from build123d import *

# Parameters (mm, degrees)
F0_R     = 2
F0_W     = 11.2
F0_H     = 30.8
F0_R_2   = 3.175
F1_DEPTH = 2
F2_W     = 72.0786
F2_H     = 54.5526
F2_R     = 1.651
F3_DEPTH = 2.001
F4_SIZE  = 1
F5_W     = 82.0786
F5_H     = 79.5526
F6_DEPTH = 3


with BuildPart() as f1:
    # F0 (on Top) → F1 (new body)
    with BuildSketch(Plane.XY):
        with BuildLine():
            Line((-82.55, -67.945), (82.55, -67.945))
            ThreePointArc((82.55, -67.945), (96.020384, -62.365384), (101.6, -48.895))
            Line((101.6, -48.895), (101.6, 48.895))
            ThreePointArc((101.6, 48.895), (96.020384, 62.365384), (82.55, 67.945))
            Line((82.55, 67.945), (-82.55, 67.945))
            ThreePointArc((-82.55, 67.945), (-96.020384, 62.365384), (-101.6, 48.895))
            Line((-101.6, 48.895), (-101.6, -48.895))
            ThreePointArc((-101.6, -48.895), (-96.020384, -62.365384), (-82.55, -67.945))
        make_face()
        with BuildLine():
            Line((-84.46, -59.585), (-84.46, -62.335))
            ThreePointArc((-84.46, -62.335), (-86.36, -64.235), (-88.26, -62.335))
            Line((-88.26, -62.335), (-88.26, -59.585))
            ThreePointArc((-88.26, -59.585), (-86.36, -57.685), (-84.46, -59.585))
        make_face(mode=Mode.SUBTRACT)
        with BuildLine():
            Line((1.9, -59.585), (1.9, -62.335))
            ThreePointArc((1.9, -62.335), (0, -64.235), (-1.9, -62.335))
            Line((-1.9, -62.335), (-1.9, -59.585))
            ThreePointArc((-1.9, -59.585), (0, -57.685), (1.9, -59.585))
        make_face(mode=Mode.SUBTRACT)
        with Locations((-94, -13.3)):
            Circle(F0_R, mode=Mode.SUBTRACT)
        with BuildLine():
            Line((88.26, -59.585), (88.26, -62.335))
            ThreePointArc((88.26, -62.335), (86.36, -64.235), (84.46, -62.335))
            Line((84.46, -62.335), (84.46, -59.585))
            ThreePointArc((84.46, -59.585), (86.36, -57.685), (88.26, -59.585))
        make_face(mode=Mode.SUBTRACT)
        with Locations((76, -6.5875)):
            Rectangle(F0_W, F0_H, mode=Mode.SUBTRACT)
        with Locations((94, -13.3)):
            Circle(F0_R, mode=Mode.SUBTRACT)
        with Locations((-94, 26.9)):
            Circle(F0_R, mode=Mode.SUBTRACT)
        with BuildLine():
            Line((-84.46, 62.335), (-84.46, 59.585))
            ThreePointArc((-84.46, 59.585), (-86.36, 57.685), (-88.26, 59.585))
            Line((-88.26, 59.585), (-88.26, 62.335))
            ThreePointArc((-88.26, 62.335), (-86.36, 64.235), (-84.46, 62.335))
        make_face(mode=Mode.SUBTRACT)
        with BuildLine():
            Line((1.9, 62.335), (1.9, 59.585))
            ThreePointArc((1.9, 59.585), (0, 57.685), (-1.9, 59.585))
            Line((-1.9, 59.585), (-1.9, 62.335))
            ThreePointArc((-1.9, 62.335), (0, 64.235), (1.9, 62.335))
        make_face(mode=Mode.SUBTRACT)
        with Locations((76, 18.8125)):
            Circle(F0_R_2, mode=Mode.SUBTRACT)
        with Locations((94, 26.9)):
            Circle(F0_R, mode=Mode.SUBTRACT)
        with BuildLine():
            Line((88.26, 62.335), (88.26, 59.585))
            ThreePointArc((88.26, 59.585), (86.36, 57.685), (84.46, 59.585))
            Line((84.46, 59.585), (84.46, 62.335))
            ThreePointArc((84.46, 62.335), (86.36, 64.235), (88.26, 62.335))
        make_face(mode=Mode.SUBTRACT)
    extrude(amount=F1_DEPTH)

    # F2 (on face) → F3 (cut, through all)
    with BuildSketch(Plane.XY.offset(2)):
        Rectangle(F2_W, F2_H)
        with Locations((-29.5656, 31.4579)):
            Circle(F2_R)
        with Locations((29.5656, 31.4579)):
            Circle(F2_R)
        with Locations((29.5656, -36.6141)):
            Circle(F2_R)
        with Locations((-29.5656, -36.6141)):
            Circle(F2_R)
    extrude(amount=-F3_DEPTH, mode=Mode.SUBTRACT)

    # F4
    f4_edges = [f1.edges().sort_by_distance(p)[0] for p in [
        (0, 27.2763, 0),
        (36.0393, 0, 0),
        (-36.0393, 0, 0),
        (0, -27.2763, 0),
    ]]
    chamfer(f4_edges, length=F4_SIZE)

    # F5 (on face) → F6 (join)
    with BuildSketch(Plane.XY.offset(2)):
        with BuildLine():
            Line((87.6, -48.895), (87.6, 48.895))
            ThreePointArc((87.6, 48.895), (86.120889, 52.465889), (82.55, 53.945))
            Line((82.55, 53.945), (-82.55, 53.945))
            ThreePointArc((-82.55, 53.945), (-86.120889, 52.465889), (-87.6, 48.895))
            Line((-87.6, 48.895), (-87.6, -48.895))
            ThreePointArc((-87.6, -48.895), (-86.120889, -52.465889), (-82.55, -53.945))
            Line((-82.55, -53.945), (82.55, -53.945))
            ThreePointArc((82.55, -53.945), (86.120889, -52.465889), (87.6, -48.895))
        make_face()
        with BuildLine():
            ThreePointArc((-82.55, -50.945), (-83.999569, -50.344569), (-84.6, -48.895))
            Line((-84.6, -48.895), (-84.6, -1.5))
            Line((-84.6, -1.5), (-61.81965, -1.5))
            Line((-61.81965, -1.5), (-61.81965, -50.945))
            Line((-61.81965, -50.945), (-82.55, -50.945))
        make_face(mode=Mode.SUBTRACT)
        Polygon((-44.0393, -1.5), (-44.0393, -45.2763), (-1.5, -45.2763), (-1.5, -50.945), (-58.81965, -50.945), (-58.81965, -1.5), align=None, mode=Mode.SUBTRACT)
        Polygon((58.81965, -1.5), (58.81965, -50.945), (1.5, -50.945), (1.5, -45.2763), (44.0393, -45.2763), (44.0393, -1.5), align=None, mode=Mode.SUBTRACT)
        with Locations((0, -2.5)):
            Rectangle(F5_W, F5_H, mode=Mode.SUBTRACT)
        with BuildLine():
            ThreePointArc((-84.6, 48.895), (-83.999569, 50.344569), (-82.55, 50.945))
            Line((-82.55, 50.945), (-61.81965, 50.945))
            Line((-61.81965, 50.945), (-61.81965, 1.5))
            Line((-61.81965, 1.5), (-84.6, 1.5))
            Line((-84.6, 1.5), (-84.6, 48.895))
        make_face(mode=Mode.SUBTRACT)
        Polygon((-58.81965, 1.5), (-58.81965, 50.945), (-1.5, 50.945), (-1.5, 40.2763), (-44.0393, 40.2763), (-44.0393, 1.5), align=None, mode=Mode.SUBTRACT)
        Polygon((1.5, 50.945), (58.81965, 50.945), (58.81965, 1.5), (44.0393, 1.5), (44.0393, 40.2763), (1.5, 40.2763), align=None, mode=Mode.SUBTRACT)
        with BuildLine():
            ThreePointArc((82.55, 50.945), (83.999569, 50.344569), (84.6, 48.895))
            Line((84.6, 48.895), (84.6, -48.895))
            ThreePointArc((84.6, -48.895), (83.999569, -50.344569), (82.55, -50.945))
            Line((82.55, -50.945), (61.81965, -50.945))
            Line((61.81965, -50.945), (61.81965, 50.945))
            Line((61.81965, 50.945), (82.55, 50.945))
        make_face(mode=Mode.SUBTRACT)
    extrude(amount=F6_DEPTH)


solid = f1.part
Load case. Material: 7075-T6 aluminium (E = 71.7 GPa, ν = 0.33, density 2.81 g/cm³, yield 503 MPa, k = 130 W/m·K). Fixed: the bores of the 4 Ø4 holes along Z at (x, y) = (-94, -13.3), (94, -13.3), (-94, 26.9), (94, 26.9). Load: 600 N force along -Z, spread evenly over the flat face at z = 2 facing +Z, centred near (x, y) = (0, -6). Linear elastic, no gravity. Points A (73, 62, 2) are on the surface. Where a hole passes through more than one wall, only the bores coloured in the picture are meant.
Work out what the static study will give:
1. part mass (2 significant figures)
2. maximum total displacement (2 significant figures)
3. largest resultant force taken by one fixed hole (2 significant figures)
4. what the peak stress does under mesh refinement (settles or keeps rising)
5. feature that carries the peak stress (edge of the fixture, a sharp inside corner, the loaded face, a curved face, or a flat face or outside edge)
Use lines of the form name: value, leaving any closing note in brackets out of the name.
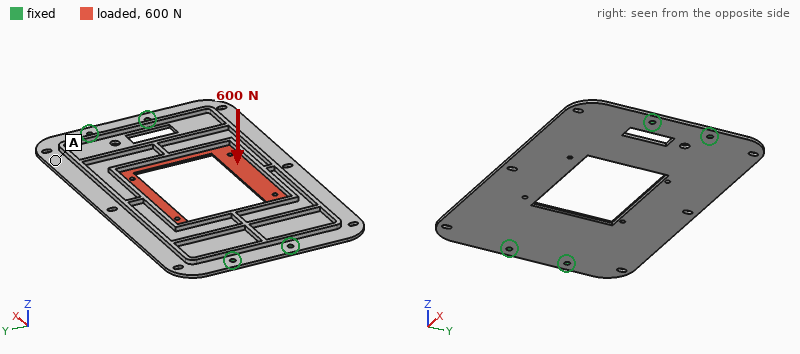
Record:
part mass: 160 g
maximum total displacement: 2.5 mm
largest resultant force taken by one fixed hole: 550 N
what the peak stress does under mesh refinement: keeps rising
feature that carries the peak stress: edge of the fixture
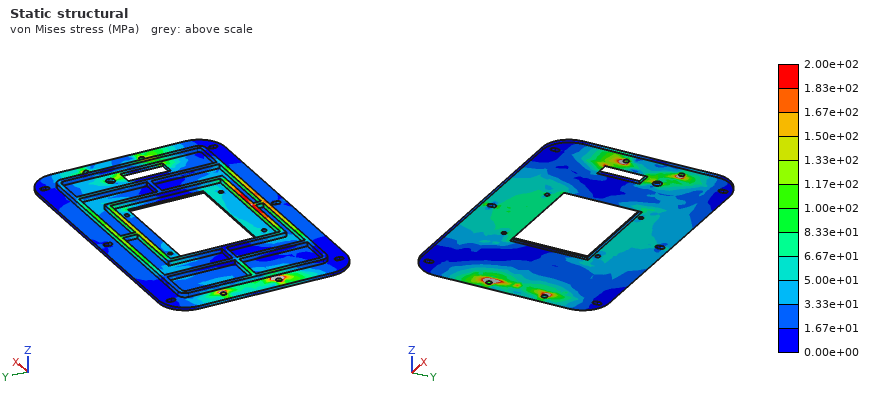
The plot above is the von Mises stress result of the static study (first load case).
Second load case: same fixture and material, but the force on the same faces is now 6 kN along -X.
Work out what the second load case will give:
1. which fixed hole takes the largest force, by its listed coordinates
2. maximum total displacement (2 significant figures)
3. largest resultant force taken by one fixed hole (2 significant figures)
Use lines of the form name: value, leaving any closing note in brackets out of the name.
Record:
which fixed hole takes the largest force, by its listed coordinates: (-94, -13.3)
maximum total displacement: 68 µm
largest resultant force taken by one fixed hole: 2.2 kN
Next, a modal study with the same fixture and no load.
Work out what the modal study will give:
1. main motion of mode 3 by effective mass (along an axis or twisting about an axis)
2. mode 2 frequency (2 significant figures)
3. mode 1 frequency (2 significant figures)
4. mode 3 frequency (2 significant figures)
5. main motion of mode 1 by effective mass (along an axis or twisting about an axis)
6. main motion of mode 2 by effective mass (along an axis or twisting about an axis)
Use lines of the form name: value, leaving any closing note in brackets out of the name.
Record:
main motion of mode 3 by effective mass: twisting about Y
mode 2 frequency: 380 Hz
mode 1 frequency: 320 Hz
mode 3 frequency: 720 Hz
main motion of mode 1 by effective mass: along Z
main motion of mode 2 by effective mass: along Z
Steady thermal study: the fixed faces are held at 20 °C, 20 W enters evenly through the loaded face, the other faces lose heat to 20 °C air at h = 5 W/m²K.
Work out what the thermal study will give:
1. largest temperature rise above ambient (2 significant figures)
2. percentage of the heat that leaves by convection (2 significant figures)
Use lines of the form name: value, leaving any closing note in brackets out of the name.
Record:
largest temperature rise above ambient: 33 K
percentage of the heat that leaves by convection: 20 %
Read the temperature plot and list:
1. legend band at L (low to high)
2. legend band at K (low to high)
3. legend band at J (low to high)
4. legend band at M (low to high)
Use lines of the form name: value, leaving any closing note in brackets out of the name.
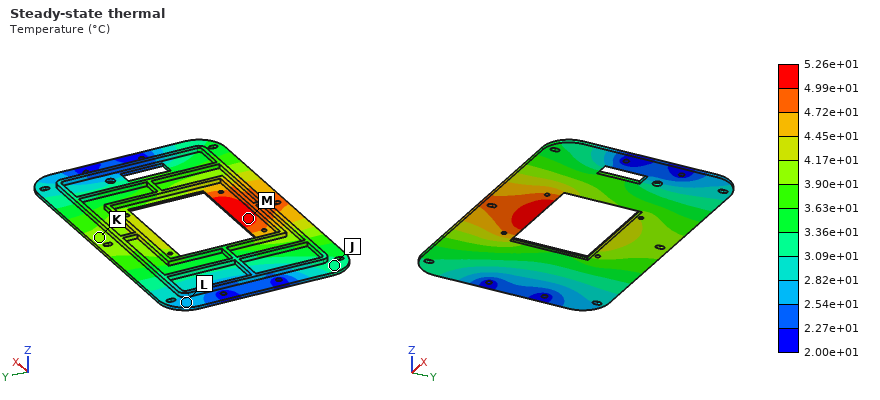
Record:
legend band at L: 2.54e+01 to 2.82e+01 °C
legend band at K: 3.90e+01 to 4.17e+01 °C
legend band at J: 3.09e+01 to 3.36e+01 °C
legend band at M: 4.99e+01 to 5.26e+01 °C
